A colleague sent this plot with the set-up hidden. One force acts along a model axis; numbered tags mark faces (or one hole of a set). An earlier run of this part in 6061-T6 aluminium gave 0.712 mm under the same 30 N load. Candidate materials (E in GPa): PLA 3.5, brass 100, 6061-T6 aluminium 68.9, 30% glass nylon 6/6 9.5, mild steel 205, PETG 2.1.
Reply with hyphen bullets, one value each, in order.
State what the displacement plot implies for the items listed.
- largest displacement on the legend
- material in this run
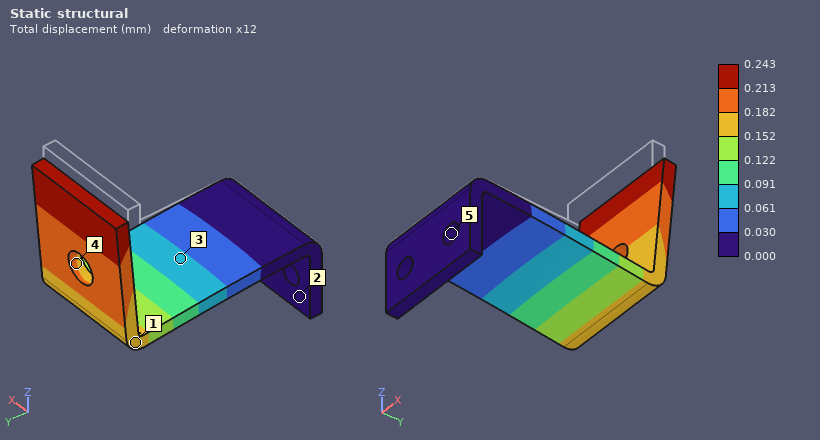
- 0.243 mm
- mild steel
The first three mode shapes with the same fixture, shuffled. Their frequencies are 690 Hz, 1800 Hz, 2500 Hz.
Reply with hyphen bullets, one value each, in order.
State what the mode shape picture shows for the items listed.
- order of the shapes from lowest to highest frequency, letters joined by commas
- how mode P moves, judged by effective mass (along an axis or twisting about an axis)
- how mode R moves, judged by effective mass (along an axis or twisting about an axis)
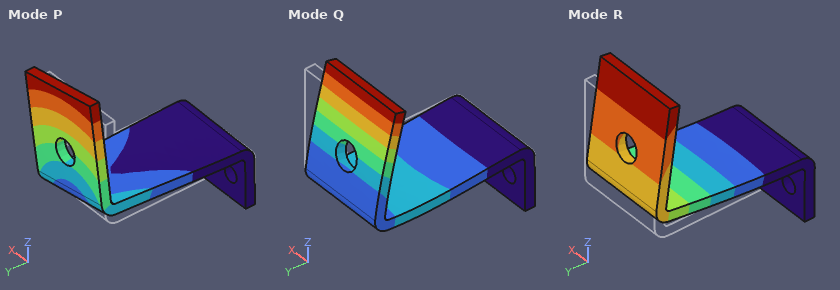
- R, P, Q
- along X
- along Z
